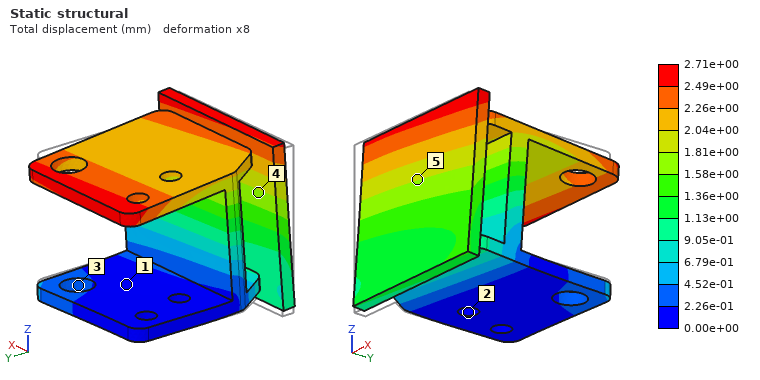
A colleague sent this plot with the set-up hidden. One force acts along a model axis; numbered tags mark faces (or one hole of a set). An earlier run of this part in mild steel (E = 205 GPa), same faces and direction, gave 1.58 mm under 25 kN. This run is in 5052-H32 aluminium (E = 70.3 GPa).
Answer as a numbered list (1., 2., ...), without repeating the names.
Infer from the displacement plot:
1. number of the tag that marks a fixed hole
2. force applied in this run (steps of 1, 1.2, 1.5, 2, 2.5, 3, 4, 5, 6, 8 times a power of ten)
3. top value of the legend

1. 2
2. 15 kN
3. 2.71e+00 mm
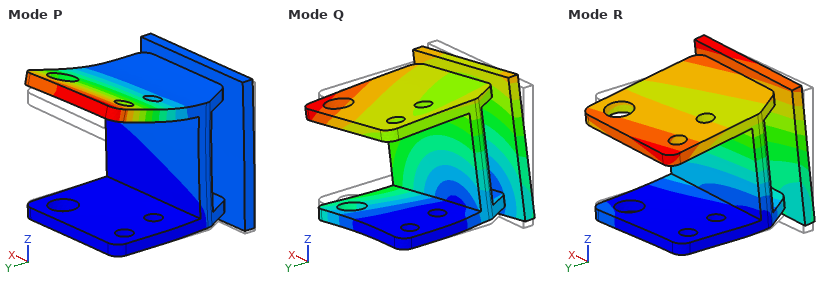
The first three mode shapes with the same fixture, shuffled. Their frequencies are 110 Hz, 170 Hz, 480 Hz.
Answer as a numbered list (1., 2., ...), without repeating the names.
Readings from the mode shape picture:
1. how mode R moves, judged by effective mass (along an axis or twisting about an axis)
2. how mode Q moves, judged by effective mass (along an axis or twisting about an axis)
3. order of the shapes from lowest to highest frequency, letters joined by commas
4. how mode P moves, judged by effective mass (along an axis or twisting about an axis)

1. along Y
2. along X
3. R, Q, P
4. along Z
